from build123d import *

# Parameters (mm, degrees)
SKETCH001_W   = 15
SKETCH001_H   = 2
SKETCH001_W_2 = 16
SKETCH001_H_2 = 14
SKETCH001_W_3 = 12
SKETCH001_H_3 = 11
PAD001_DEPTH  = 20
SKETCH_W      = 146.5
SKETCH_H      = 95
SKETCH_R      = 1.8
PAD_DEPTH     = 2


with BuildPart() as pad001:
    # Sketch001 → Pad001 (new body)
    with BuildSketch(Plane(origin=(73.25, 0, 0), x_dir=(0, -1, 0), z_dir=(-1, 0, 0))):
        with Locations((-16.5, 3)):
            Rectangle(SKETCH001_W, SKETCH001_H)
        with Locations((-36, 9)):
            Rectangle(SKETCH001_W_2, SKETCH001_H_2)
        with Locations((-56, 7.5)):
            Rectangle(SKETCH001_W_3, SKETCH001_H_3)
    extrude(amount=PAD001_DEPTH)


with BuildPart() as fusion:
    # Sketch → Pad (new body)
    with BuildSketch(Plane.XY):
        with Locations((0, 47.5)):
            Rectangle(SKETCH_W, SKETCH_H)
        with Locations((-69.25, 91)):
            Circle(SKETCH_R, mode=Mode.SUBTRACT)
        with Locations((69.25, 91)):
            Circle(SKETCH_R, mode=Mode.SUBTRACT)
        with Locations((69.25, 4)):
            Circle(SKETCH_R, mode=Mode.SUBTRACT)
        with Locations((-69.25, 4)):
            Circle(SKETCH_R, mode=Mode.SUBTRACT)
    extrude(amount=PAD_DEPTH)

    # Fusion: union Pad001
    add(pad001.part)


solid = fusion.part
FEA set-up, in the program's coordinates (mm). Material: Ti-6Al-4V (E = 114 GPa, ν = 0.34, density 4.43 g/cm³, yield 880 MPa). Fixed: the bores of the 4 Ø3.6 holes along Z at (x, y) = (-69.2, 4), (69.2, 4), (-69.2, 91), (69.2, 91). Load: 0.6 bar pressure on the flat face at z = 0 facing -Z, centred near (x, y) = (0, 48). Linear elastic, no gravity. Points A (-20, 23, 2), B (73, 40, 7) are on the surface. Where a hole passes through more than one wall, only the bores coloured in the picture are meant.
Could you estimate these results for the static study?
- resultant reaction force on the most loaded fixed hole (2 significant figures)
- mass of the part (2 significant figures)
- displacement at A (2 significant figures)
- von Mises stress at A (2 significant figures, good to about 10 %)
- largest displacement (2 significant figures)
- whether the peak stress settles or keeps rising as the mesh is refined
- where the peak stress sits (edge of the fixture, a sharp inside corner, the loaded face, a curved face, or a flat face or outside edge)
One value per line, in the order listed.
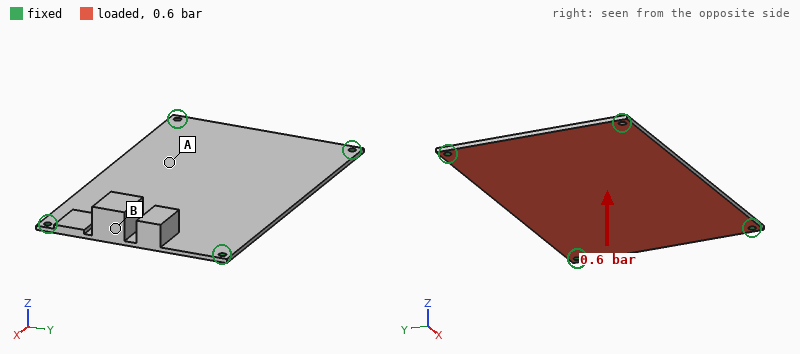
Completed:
240 N
160 g
1.0 mm
69 MPa
1.2 mm
keeps rising
edge of the fixture
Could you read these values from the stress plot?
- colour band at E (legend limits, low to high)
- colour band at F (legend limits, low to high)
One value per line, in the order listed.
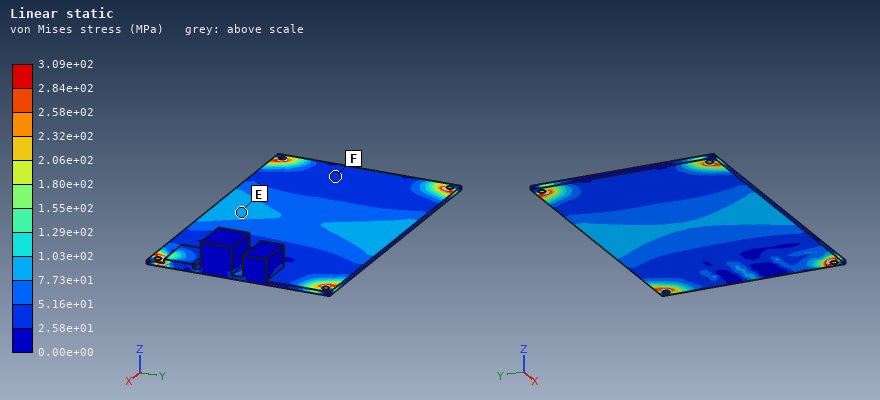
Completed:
7.73e+01 to 1.03e+02 MPa
2.58e+01 to 5.16e+01 MPa
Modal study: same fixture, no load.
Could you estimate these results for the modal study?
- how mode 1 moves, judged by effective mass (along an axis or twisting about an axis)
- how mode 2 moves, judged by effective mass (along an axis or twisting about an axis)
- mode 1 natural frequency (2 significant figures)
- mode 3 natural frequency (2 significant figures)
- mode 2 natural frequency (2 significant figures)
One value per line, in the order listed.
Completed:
along Z
twisting about X
430 Hz
900 Hz
790 Hz
